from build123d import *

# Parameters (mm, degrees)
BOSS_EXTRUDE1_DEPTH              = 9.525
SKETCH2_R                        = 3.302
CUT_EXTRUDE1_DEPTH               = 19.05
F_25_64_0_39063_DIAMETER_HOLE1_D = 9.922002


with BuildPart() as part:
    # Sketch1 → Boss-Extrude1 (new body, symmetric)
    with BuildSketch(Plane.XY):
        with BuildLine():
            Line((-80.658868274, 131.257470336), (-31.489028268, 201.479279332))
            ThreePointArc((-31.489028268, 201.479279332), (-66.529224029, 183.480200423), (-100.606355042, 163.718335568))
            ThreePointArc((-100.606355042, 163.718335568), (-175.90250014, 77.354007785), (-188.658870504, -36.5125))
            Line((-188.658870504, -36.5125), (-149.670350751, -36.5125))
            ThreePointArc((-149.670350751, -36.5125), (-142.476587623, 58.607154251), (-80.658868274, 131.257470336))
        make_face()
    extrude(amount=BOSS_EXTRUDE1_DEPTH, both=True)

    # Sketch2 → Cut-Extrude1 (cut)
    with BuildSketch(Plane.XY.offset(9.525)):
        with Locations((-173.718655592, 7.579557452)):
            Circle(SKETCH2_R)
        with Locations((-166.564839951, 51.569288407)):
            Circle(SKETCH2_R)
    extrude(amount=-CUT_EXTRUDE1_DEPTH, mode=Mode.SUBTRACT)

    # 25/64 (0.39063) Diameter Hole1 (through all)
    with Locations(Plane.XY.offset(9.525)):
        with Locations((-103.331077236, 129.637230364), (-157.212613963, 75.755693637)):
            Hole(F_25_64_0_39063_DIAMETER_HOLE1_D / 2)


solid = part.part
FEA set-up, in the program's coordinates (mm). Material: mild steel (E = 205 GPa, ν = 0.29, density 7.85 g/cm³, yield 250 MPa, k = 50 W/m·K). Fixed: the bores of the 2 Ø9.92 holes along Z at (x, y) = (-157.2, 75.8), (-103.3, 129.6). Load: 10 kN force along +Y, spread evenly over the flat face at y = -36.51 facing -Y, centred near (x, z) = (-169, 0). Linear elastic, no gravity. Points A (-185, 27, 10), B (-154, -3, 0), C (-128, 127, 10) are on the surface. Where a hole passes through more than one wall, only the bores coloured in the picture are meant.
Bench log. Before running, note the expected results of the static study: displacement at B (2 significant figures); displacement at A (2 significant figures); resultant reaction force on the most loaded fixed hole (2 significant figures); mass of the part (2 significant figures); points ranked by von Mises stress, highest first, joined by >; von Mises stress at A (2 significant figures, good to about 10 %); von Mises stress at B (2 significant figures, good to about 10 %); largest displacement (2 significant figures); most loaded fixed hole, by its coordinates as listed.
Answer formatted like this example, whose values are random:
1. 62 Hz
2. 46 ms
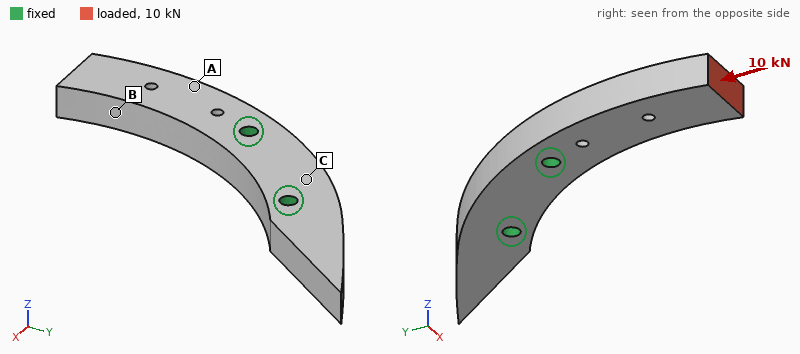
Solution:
1. 20 µm
2. 16 µm
3. 10 kN
4. 1.4 kg
5. B > A > C
6. 12 MPa
7. 25 MPa
8. 29 µm
9. (-157.2, 75.8)
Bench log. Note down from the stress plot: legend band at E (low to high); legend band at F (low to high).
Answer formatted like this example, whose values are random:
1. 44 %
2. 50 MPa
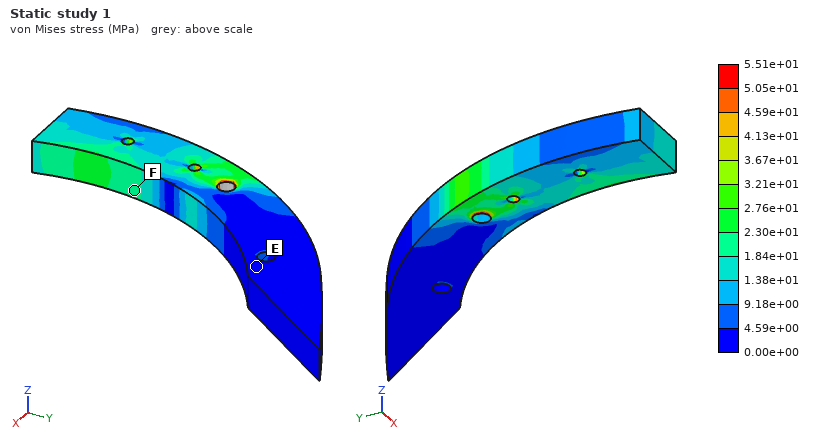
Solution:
1. 0.00e+00 to 4.59e+00 MPa
2. 1.84e+01 to 2.30e+01 MPa
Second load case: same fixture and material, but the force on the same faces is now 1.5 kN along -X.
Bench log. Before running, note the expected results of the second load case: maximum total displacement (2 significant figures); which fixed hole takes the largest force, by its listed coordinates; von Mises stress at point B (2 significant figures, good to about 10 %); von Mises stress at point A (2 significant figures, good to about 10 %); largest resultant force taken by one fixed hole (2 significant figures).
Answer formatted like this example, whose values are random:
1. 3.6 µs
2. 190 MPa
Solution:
1. 63 µm
2. (-157.2, 75.8)
3. 11 MPa
4. 14 MPa
5. 2.8 kN
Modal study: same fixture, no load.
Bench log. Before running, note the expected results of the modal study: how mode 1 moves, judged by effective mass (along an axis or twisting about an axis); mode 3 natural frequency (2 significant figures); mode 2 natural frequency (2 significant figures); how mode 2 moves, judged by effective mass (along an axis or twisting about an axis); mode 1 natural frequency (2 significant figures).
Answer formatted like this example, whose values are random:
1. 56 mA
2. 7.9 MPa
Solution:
1. along Z
2. 2700 Hz
3. 1800 Hz
4. along X
5. 1200 Hz
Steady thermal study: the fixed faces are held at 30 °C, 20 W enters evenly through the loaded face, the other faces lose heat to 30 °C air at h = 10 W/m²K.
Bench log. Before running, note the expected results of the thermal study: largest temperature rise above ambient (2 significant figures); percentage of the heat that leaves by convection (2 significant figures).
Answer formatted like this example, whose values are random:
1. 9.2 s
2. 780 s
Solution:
1. 59 K
2. 19 %
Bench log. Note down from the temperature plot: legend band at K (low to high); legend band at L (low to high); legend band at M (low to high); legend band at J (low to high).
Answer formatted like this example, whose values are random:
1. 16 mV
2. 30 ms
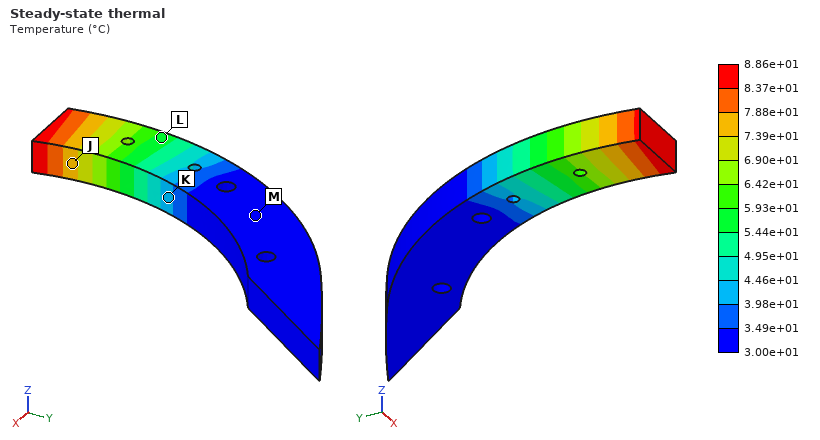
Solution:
1. 3.98e+01 to 4.46e+01 °C
2. 5.44e+01 to 5.93e+01 °C
3. 3.00e+01 to 3.49e+01 °C
4. 7.39e+01 to 7.88e+01 °C
